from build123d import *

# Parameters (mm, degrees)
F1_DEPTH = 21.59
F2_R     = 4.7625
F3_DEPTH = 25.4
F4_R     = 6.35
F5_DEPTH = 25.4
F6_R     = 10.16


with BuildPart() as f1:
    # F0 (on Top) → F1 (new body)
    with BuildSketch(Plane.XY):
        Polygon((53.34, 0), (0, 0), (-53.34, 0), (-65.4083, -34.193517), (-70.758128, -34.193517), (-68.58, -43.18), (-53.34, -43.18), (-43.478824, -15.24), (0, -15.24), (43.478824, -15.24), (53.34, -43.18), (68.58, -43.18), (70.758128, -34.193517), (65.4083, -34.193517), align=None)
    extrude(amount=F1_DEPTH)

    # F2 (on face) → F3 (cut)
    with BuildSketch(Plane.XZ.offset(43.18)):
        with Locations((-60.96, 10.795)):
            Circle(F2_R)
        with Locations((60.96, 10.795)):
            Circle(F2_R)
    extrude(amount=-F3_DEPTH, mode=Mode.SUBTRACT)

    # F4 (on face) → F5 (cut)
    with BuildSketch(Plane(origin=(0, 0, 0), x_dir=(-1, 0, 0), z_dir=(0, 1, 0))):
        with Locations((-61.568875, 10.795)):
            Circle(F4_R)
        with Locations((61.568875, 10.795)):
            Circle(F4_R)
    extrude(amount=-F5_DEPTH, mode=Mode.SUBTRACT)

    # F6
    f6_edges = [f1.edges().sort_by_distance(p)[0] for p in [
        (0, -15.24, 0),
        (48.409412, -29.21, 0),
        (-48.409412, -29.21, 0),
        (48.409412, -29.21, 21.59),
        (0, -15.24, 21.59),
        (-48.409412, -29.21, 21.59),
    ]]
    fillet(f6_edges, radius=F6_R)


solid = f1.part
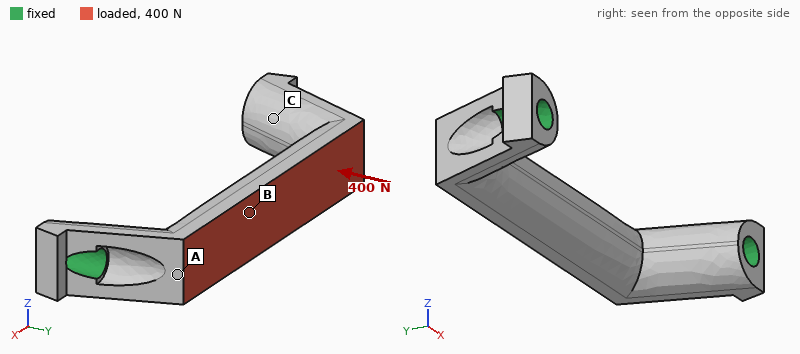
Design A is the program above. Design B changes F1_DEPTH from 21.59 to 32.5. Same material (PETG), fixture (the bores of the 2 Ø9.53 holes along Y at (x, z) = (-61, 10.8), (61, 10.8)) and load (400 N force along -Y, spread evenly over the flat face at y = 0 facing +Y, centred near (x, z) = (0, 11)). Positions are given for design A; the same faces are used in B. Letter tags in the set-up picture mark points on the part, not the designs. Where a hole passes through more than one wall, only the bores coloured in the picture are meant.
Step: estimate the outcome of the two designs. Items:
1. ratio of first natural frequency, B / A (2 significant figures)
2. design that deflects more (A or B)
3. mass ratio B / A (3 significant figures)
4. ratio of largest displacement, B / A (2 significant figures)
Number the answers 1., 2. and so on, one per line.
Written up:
1. 1.1
2. A
3. 1.62
4. 0.67
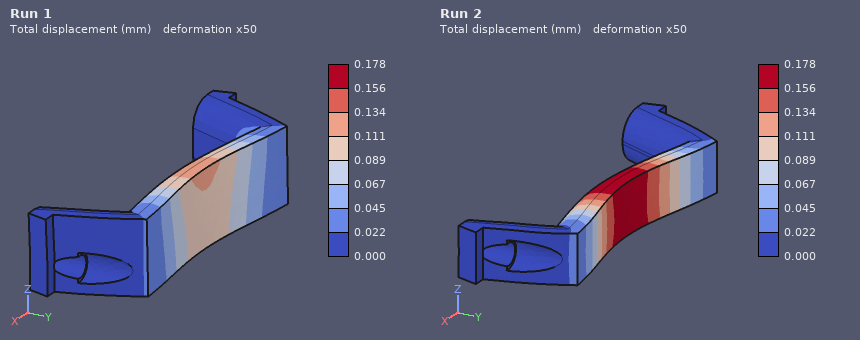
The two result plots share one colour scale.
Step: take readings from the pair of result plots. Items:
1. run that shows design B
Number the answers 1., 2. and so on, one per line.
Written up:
1. Run 1
